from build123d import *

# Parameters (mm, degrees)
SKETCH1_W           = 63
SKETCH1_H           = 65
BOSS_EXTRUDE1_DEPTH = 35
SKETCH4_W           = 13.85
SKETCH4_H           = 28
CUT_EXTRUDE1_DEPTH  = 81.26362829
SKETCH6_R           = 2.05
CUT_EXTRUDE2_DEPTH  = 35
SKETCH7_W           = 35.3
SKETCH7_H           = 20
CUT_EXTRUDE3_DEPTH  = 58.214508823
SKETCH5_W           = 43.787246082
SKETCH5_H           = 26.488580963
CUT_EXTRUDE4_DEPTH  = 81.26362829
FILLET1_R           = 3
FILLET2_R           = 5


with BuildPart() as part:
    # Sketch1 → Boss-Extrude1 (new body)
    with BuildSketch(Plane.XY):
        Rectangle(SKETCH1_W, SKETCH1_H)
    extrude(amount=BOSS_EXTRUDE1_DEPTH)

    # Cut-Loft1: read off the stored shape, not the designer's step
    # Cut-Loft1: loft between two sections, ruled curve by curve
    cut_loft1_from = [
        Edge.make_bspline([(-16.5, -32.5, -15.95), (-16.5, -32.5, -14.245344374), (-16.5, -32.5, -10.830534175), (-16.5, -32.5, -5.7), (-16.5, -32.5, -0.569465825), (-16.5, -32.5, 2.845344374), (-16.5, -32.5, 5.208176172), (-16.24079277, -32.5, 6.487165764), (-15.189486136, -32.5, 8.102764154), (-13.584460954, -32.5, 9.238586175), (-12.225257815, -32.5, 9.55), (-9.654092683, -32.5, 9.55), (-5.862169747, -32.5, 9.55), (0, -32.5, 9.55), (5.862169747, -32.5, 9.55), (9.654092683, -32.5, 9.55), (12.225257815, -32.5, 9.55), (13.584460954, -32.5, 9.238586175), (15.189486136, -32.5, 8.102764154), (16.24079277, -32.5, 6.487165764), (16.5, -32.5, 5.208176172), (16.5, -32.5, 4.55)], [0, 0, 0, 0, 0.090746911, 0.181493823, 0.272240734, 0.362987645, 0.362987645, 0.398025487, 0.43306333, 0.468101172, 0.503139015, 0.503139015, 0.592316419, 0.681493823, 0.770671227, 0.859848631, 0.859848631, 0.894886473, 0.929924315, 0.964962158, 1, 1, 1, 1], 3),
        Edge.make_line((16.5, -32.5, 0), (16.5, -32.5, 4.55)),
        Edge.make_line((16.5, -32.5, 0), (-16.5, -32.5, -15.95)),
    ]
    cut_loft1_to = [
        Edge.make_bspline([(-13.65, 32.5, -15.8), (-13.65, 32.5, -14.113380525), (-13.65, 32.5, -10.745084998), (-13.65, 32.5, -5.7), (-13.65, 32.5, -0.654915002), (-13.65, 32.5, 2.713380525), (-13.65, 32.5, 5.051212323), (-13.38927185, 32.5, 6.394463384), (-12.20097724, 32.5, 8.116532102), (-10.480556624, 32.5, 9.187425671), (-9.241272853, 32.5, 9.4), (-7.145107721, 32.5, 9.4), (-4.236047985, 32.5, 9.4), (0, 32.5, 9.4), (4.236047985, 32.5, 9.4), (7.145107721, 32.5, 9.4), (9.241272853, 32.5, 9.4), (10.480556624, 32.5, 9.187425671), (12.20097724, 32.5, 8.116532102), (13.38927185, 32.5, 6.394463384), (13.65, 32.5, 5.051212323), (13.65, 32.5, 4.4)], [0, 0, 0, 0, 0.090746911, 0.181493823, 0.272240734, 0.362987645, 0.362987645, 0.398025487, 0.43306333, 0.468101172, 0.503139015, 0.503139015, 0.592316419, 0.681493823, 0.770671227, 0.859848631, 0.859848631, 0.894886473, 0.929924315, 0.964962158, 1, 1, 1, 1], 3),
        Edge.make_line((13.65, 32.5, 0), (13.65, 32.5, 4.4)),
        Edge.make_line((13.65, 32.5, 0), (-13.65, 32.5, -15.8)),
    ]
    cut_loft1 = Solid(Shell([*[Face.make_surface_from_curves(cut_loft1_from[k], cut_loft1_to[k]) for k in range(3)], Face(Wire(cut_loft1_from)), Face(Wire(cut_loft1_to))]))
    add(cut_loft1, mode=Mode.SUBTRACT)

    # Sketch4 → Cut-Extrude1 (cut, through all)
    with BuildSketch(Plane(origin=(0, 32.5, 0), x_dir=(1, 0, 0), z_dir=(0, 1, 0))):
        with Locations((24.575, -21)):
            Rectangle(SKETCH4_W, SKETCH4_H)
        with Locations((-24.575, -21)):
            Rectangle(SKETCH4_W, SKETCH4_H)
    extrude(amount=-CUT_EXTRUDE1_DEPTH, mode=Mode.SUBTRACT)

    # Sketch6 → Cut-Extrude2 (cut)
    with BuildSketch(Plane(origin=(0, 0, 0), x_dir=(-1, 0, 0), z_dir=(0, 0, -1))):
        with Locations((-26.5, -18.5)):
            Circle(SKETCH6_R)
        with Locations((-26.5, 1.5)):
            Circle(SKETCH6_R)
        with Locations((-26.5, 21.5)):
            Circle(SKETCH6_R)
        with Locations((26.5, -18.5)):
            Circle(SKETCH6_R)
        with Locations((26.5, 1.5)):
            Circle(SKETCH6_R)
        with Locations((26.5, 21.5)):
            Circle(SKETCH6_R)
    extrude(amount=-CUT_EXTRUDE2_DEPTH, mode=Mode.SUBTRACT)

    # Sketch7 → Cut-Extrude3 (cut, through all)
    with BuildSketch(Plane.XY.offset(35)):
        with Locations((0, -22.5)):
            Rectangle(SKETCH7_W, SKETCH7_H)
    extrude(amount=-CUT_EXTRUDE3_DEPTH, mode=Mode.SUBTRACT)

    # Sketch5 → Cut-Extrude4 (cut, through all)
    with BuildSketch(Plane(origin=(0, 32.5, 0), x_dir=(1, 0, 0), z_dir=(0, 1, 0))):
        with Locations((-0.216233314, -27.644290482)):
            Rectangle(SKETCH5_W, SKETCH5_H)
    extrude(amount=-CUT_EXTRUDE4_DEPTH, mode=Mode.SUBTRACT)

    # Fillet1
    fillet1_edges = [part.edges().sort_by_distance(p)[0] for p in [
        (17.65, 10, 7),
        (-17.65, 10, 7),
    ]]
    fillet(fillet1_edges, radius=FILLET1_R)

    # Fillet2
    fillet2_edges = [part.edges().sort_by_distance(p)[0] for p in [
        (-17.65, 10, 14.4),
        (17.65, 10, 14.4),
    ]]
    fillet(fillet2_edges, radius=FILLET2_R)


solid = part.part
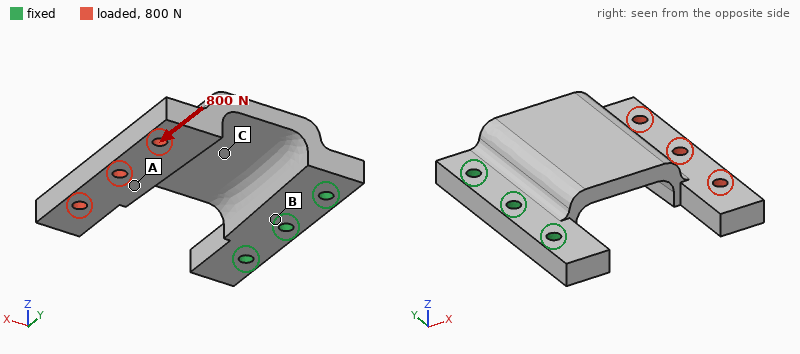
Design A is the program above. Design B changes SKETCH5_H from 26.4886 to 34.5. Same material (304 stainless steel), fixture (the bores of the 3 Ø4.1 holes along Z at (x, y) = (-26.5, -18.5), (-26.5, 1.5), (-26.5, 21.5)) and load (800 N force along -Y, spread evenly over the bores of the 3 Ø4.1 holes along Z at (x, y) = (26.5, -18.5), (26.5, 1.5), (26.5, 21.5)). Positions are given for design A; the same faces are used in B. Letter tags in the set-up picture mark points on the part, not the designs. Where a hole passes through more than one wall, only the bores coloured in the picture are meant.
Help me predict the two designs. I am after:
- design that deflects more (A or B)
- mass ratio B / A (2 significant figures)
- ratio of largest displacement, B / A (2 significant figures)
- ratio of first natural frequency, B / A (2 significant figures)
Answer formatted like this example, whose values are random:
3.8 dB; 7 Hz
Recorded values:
B; 0.73; 18; 0.15
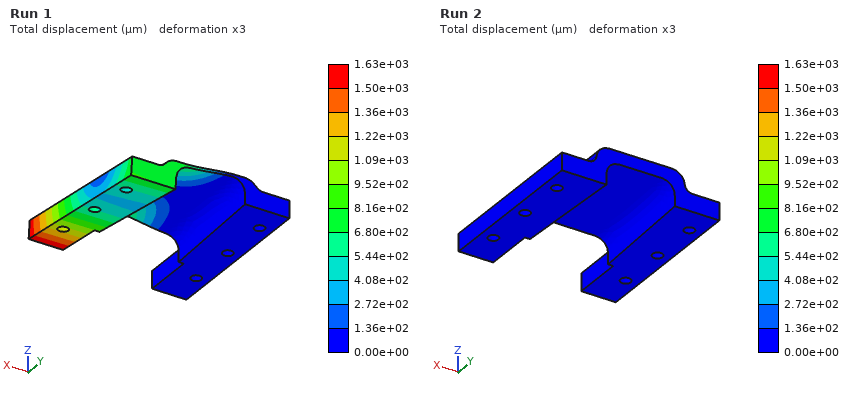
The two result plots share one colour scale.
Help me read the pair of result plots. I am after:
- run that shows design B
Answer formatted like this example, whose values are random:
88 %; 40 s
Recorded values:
Run 1
